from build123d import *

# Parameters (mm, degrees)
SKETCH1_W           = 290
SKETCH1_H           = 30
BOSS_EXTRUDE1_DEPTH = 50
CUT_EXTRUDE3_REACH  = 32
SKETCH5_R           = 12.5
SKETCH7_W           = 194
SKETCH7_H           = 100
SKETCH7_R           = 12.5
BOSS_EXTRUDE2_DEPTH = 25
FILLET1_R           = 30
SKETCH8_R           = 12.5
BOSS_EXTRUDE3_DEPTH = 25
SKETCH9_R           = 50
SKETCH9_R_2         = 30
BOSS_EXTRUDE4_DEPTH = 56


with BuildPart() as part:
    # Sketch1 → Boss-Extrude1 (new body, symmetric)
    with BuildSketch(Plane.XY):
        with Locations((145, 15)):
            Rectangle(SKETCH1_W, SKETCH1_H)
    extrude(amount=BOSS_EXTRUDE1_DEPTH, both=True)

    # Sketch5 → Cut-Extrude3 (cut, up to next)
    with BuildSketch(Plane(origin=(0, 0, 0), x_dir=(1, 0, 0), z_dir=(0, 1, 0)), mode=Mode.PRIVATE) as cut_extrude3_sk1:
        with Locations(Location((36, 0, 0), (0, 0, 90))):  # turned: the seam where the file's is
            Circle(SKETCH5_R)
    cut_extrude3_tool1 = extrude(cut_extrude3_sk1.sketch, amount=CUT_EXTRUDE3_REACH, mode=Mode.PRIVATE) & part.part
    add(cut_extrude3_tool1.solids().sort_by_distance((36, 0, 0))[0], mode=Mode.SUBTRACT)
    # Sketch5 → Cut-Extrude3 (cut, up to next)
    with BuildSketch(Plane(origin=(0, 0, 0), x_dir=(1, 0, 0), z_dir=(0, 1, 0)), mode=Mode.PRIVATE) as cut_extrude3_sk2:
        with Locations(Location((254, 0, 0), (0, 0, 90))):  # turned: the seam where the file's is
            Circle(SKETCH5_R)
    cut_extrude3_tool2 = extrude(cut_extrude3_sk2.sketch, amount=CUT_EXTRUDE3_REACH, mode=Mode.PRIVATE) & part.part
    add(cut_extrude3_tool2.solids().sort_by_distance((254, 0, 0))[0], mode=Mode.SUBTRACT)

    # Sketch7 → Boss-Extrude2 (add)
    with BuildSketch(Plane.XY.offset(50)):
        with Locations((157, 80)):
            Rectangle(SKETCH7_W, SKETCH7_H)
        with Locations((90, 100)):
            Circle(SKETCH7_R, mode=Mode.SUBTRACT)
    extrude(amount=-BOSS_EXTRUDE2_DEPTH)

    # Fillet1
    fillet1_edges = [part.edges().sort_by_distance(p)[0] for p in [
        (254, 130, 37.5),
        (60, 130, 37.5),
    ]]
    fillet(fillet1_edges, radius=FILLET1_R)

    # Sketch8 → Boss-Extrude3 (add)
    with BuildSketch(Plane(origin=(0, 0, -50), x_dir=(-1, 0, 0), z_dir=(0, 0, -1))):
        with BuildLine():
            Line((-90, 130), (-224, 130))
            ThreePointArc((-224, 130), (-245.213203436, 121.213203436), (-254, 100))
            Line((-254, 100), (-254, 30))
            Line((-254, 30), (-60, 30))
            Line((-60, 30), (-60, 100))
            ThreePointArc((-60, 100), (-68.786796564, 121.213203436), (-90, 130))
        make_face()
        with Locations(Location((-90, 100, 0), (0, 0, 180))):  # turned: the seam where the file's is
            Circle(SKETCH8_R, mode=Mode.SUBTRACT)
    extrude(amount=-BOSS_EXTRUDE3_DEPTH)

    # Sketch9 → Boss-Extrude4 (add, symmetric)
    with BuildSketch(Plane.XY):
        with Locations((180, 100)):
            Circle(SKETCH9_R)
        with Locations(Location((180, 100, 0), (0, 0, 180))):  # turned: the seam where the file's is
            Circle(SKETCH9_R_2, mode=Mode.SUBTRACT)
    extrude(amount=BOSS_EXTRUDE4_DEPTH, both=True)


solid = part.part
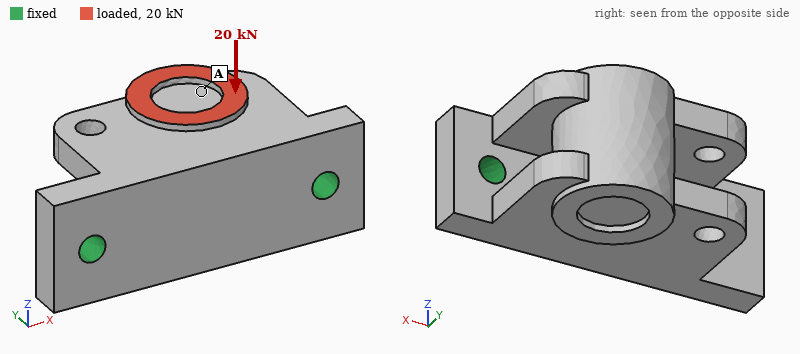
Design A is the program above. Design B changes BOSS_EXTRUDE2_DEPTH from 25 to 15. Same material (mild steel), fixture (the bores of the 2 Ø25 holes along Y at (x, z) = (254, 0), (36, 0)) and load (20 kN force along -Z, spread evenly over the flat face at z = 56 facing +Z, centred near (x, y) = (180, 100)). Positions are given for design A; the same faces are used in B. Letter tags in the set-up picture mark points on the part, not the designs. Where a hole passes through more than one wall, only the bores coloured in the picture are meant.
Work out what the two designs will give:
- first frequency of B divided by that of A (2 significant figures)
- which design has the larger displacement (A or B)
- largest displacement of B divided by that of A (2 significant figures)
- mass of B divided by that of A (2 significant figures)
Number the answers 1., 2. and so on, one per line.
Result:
1. 1.00
2. B
3. 1.1
4. 0.93
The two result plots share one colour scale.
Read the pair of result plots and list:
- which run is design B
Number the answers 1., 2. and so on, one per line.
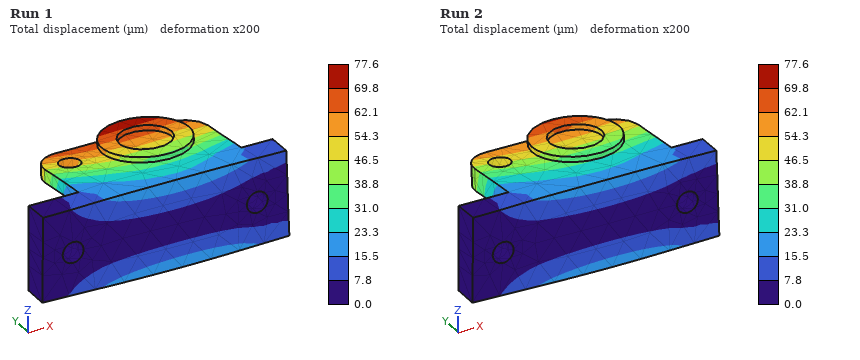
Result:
1. Run 1
